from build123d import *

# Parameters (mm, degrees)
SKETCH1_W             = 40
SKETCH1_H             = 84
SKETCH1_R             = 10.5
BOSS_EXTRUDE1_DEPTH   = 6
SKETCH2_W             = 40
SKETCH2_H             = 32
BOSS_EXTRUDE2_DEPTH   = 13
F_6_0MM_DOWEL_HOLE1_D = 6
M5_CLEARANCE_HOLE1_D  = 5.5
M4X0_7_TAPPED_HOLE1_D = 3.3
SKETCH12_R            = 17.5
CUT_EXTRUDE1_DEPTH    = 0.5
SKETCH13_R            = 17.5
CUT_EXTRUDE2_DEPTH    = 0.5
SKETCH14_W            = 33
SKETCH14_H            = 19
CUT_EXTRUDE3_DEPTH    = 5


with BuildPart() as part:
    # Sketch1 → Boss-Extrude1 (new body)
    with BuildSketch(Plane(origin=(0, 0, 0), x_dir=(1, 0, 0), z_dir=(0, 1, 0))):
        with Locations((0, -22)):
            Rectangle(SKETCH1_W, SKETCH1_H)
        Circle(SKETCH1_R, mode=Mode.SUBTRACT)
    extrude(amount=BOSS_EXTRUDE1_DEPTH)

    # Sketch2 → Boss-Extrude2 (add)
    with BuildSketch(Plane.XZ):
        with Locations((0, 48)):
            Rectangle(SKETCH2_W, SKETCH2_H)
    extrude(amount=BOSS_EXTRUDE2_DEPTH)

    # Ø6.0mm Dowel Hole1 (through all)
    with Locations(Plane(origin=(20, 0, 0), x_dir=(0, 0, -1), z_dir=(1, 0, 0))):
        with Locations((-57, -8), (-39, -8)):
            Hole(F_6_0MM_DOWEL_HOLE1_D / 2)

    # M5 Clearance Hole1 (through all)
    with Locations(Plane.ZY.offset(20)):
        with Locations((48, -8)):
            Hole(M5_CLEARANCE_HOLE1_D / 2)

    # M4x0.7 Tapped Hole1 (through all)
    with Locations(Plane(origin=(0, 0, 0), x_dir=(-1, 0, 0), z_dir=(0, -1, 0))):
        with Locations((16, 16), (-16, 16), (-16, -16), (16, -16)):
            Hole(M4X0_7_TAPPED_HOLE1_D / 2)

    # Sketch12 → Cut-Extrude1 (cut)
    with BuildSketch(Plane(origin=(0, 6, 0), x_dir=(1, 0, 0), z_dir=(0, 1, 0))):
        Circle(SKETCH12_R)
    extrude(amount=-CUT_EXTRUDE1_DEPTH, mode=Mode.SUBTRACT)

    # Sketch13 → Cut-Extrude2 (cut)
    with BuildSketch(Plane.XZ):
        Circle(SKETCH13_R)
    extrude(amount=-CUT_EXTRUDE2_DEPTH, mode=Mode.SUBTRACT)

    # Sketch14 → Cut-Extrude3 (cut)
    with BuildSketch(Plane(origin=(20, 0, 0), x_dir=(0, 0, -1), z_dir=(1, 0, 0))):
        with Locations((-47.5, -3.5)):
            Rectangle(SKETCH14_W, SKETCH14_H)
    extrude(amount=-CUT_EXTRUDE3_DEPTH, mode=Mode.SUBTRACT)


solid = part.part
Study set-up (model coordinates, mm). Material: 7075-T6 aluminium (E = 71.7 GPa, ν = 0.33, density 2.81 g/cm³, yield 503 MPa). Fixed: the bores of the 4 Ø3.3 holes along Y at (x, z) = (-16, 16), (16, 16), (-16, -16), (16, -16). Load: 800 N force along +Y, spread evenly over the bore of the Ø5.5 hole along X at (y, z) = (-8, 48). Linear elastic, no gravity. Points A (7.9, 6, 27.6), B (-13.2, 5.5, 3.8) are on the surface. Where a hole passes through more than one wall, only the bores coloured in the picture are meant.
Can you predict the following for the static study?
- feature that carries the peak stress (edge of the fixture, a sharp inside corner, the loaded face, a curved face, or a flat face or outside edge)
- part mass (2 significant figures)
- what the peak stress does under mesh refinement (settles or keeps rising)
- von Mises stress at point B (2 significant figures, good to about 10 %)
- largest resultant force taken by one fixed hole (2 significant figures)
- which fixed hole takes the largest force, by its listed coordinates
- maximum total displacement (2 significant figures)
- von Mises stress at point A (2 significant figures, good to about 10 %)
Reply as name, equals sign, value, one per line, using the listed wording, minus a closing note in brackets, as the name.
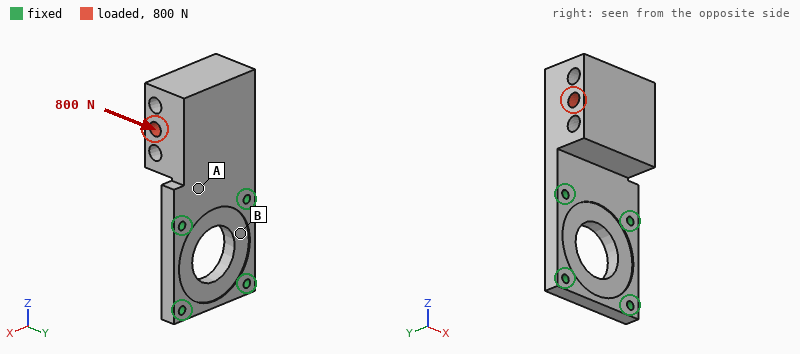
feature that carries the peak stress = edge of the fixture
part mass = 79 g
what the peak stress does under mesh refinement = keeps rising
von Mises stress at point B = 16 MPa
largest resultant force taken by one fixed hole = 530 N
which fixed hole takes the largest force, by its listed coordinates = (-16, 16)
maximum total displacement = 0.37 mm
von Mises stress at point A = 68 MPa
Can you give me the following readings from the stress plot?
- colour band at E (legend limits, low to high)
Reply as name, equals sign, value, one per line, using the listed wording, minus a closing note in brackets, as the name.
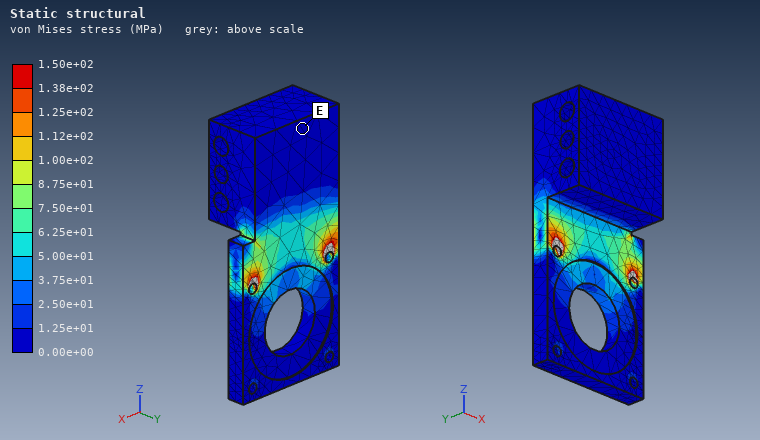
colour band at E = 0.00e+00 to 1.25e+01 MPa
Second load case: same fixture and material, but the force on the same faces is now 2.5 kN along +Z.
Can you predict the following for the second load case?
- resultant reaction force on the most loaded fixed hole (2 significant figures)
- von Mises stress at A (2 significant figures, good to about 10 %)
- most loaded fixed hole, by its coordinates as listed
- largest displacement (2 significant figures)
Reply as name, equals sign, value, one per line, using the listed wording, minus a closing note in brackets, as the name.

resultant reaction force on the most loaded fixed hole = 1.4 kN
von Mises stress at A = 100 MPa
most loaded fixed hole, by its coordinates as listed = (-16, 16)
largest displacement = 0.51 mm
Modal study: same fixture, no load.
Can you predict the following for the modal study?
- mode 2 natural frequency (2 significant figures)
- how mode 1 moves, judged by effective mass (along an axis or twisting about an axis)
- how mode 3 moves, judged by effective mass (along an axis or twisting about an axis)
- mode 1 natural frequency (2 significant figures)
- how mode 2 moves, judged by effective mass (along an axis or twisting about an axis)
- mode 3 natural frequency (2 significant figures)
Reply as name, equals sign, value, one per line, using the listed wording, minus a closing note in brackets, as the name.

mode 2 natural frequency = 5000 Hz
how mode 1 moves, judged by effective mass = along Y
how mode 3 moves, judged by effective mass = along X
mode 1 natural frequency = 1200 Hz
how mode 2 moves, judged by effective mass = along X
mode 3 natural frequency = 7100 Hz
